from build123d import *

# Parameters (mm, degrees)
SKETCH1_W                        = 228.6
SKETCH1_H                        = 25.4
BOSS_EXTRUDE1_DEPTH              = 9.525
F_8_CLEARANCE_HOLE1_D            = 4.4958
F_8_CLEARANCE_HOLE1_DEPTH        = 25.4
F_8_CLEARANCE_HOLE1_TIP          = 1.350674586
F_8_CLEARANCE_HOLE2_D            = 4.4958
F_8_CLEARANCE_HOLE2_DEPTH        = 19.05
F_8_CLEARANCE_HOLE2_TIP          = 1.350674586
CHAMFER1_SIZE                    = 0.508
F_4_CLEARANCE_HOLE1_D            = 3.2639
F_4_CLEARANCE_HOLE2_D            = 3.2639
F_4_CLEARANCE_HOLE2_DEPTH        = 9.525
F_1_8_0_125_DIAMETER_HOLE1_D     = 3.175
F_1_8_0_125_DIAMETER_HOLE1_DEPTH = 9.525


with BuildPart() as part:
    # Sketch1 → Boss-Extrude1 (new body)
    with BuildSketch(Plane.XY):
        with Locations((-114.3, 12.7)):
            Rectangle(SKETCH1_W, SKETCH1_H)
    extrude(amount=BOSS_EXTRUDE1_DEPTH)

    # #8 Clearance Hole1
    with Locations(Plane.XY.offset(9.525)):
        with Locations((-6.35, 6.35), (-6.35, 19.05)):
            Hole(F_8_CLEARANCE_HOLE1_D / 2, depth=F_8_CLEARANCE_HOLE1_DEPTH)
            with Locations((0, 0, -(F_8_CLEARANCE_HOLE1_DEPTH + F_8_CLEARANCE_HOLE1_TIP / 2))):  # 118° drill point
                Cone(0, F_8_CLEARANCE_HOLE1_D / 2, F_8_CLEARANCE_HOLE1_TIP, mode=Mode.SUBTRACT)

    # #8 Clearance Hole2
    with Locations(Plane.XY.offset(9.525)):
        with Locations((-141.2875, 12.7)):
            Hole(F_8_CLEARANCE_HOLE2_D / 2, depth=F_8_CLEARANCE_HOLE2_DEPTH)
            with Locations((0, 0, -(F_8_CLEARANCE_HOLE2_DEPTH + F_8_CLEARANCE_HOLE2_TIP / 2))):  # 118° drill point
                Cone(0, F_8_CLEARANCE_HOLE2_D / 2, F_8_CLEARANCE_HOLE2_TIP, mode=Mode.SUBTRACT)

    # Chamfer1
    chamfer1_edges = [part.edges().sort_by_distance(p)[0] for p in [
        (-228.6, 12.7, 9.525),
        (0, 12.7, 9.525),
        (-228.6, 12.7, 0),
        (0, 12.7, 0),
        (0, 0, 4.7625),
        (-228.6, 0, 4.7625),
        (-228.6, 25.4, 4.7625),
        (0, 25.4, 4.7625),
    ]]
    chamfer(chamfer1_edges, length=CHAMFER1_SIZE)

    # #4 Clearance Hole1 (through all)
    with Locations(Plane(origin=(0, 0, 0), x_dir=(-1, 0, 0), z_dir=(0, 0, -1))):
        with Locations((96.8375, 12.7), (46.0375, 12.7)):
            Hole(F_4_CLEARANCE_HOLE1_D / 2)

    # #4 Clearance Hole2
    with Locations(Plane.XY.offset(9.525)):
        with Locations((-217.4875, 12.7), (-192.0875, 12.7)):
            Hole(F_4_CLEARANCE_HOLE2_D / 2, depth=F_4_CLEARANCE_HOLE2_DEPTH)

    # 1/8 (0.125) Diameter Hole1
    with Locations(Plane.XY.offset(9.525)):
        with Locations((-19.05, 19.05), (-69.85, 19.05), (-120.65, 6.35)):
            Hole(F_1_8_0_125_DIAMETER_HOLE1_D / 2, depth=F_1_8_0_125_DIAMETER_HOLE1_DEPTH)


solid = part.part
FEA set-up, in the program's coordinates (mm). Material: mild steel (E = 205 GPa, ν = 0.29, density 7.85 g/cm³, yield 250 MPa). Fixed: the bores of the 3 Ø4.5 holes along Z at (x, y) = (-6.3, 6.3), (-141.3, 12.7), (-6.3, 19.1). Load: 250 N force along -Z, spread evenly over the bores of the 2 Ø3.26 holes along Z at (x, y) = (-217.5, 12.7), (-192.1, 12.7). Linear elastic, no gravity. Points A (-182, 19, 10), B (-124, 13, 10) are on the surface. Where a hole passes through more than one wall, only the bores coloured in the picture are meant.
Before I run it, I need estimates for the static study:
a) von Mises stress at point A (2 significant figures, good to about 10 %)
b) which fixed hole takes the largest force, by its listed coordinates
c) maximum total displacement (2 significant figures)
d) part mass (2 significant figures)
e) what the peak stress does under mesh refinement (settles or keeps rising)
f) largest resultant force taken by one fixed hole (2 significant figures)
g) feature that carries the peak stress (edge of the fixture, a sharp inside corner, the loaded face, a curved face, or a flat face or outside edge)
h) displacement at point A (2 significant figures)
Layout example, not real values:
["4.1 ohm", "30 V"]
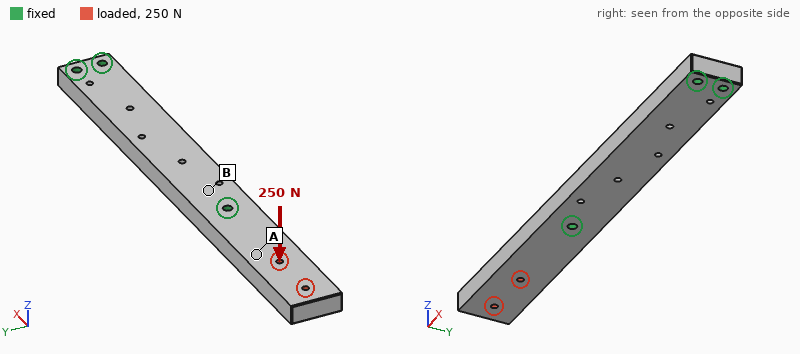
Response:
["15 MPa", "(-141.3, 12.7)", "98 µm", "430 g", "keeps rising", "260 N", "edge of the fixture", "31 µm"]
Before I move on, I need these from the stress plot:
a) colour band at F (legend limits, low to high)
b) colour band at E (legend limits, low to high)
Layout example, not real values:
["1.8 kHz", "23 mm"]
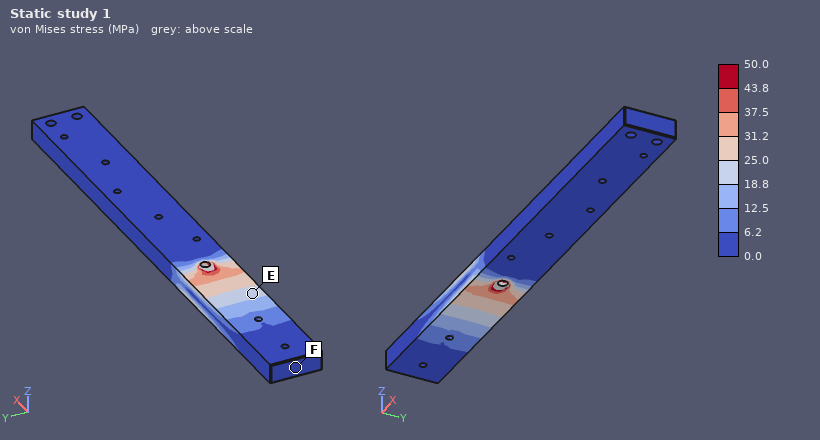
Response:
["0.0 to 6.2 MPa", "18.8 to 25.0 MPa"]
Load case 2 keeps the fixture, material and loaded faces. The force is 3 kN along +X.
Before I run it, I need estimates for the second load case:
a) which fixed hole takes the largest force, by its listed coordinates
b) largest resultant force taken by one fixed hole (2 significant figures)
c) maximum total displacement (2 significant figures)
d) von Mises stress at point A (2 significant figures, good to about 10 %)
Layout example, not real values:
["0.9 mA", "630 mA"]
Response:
["(-141.3, 12.7)", "2.9 kN", "4.6 µm", "13 MPa"]
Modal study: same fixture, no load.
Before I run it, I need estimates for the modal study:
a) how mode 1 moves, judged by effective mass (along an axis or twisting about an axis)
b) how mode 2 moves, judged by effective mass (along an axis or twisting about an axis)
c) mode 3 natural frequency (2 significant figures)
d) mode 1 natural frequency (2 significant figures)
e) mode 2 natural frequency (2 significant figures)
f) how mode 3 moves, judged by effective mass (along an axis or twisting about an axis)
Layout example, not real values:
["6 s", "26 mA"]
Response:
["along Z", "along Y", "2600 Hz", "990 Hz", "1900 Hz", "along Z"]
